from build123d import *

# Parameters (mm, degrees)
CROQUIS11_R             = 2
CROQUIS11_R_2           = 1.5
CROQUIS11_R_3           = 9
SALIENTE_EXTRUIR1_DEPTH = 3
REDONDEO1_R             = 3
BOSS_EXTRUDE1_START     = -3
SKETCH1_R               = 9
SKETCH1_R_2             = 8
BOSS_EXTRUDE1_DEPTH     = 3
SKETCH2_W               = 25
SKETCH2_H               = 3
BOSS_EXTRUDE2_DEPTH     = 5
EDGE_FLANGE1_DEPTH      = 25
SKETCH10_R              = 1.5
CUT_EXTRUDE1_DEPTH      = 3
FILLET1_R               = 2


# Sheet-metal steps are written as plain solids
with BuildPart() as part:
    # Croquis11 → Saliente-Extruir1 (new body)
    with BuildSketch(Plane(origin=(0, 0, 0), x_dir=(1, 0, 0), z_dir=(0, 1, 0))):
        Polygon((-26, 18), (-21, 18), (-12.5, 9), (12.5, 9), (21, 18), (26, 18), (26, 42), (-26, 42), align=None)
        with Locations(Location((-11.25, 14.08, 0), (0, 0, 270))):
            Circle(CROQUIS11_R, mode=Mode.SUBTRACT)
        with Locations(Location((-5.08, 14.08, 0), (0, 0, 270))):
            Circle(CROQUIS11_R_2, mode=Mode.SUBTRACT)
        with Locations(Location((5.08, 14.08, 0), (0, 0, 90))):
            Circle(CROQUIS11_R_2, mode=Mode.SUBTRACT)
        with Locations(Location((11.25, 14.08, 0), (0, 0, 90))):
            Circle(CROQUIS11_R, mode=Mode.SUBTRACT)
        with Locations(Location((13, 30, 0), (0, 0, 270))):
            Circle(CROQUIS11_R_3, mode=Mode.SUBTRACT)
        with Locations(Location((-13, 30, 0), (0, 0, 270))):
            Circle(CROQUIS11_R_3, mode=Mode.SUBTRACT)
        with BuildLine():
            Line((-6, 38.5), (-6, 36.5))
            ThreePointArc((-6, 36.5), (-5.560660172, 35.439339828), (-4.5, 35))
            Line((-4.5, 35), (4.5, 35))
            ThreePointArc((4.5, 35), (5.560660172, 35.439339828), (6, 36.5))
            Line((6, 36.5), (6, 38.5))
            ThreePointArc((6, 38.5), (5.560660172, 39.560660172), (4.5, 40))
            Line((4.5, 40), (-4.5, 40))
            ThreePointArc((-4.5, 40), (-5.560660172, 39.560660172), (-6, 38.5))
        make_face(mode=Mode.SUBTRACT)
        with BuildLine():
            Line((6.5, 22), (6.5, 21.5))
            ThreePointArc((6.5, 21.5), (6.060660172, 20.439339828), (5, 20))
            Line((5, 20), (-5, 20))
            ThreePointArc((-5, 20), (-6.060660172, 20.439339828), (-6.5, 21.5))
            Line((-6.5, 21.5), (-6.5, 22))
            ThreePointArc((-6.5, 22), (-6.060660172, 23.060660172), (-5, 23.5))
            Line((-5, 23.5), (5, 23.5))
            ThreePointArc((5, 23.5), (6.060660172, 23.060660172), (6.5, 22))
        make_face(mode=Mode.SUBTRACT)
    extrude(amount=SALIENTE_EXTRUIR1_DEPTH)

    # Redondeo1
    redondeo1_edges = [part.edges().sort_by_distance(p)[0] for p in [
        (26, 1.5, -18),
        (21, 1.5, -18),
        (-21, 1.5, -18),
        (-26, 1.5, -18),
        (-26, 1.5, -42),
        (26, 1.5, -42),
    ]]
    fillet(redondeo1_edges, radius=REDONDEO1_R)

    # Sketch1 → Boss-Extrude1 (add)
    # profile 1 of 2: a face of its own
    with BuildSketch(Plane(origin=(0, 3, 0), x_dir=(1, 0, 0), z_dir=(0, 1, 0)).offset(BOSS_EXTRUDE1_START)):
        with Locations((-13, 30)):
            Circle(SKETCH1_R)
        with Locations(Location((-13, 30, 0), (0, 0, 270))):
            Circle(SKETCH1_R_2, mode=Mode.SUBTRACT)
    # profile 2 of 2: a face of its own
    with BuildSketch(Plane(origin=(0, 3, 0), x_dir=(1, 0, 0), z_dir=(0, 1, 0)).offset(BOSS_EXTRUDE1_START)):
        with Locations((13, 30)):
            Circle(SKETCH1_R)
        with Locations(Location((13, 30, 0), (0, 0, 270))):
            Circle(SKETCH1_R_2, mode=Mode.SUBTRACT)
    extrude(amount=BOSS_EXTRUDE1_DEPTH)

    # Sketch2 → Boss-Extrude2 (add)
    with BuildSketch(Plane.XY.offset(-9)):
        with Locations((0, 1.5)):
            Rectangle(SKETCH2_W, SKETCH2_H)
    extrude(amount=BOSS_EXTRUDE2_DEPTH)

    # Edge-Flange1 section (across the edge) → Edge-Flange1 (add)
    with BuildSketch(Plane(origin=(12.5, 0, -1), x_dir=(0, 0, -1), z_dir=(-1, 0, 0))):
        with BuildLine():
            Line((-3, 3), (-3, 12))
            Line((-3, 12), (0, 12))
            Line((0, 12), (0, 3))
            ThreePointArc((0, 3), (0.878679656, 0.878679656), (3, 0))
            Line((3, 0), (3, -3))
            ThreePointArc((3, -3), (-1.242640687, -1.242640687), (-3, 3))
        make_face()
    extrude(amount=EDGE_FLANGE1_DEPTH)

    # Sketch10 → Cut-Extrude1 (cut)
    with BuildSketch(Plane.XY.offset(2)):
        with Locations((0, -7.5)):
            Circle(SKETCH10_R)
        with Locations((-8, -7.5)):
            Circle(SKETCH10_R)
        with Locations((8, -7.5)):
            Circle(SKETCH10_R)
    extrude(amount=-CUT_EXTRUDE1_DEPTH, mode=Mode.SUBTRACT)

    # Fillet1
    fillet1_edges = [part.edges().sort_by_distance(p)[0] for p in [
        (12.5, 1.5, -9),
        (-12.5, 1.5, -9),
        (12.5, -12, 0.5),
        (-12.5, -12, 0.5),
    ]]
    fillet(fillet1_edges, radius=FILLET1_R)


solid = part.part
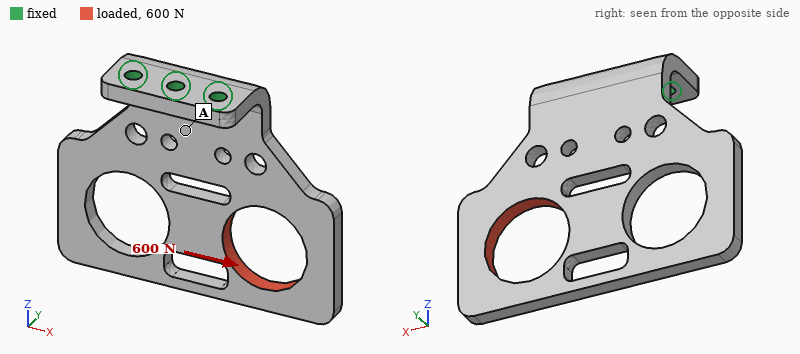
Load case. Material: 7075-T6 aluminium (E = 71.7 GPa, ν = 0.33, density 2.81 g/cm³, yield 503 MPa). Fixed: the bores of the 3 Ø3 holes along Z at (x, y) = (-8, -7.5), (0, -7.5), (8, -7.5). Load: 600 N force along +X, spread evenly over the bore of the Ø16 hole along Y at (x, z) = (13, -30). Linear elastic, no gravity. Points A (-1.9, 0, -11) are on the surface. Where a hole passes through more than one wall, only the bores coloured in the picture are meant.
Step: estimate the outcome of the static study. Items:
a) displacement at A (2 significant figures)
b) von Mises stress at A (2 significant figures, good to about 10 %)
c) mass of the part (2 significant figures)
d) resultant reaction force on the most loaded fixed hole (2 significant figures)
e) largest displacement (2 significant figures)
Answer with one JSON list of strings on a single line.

["0.095 mm", "56 MPa", "13 g", "1.0 kN", "0.47 mm"]
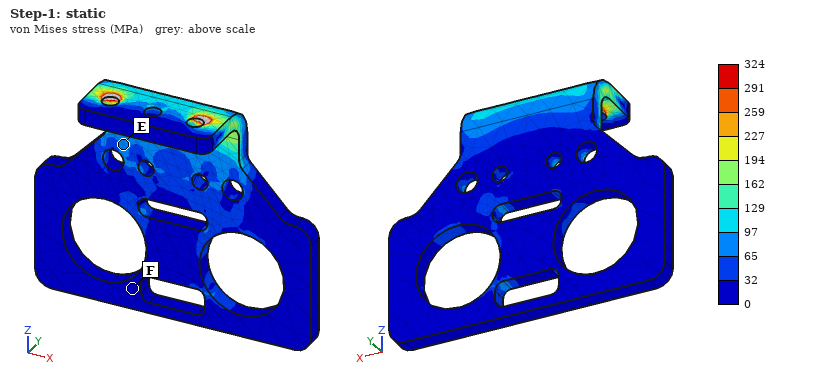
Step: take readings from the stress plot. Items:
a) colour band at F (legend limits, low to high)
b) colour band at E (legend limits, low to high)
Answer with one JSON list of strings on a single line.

["0 to 32 MPa", "65 to 97 MPa"]
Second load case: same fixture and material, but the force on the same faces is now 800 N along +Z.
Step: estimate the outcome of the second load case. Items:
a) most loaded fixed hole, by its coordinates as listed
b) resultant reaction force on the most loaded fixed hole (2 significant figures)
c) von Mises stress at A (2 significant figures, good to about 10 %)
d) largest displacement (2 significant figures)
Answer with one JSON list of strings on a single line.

["(8, -7.5)", "820 N", "29 MPa", "0.49 mm"]
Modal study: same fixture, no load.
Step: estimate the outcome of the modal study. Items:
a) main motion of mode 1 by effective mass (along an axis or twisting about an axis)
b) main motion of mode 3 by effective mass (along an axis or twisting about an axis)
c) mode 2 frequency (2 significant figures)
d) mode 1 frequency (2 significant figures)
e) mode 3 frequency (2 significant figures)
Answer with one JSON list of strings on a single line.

["along Y", "along X", "1700 Hz", "940 Hz", "2700 Hz"]
